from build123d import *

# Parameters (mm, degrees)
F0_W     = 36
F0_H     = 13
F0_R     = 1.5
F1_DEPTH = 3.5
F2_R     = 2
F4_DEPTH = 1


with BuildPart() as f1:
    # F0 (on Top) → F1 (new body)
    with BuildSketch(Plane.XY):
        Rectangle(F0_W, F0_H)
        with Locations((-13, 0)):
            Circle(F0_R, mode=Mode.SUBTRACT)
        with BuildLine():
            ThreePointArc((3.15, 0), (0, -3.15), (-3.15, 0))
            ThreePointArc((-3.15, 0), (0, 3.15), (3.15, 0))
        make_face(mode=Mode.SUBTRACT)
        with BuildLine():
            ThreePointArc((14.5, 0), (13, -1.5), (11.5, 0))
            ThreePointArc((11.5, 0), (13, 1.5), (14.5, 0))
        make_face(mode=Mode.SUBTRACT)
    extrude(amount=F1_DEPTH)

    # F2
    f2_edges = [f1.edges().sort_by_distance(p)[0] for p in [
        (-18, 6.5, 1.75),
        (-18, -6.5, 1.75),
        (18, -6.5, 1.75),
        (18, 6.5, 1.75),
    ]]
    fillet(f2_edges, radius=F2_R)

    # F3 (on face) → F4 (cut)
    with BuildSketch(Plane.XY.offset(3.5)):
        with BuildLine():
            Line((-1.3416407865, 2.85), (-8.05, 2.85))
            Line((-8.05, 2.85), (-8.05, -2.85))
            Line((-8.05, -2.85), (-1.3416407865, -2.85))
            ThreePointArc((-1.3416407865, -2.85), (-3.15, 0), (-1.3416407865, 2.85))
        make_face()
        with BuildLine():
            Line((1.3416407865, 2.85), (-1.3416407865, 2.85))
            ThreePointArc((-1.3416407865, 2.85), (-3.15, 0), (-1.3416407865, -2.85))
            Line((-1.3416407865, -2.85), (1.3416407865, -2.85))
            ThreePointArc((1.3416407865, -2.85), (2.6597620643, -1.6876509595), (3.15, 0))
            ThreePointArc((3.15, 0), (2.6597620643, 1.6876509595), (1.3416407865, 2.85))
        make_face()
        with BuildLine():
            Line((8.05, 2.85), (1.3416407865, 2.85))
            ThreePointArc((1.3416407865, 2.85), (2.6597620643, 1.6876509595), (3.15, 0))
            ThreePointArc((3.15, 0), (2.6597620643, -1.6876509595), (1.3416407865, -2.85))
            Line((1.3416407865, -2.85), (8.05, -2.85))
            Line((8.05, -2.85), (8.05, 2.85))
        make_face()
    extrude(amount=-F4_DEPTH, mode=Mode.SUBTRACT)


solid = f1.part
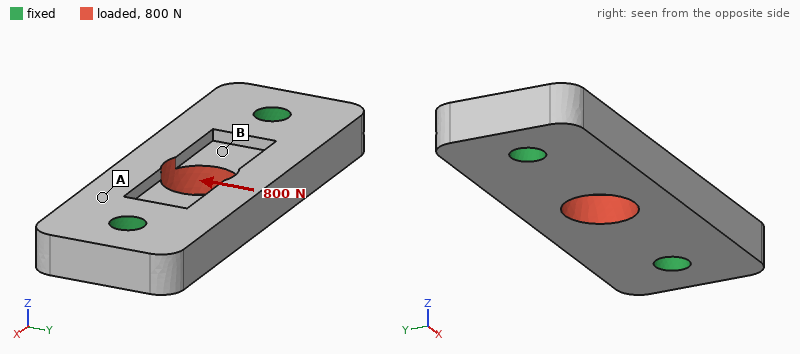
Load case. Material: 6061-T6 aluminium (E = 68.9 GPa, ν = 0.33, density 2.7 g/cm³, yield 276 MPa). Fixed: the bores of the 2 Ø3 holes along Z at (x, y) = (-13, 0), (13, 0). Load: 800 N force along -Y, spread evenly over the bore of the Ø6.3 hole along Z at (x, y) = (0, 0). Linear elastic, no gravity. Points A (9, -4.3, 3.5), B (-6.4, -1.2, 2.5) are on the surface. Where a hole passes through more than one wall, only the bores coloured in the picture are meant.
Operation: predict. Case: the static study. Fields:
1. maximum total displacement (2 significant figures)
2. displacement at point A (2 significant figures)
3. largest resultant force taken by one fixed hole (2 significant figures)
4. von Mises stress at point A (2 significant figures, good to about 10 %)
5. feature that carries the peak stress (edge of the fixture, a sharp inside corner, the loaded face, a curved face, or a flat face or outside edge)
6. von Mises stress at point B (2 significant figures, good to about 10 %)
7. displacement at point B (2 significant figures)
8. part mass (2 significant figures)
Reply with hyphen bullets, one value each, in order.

- 9.8 µm
- 3.2 µm
- 400 N
- 12 MPa
- edge of the fixture
- 31 MPa
- 5.2 µm
- 3.8 g
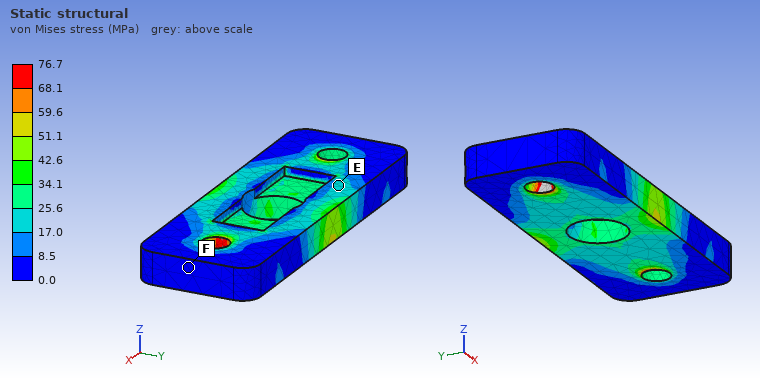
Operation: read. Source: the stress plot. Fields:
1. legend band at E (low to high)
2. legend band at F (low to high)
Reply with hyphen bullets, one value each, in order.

- 17.0 to 25.6 MPa
- 0.0 to 8.5 MPa
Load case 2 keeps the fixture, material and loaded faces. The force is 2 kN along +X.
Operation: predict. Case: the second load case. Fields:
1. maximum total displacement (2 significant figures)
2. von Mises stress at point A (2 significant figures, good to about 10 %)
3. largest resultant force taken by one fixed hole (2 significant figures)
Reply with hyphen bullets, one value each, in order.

- 6.3 µm
- 21 MPa
- 1.0 kN
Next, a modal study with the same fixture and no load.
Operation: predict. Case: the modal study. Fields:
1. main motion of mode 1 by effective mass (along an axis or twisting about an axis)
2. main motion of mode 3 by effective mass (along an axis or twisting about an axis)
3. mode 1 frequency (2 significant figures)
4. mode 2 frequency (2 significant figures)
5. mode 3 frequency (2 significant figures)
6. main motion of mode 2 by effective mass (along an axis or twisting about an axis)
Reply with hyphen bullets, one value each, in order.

- along Z
- along Y
- 25 kHz
- 28 kHz
- 43 kHz
- twisting about X
